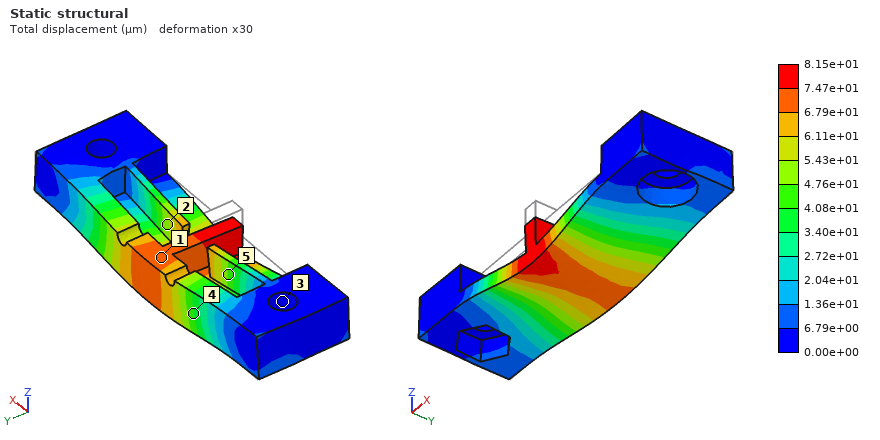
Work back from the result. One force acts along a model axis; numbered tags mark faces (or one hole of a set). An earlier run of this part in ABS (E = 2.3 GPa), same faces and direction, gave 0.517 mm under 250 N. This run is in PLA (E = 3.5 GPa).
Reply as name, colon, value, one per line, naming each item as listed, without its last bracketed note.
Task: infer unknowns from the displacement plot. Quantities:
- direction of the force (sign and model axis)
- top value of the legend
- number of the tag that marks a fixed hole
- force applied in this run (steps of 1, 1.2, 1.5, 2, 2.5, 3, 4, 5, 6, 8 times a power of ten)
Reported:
direction of the force: -Z
top value of the legend: 8.15e+01 µm
number of the tag that marks a fixed hole: 3
force applied in this run: 60 N
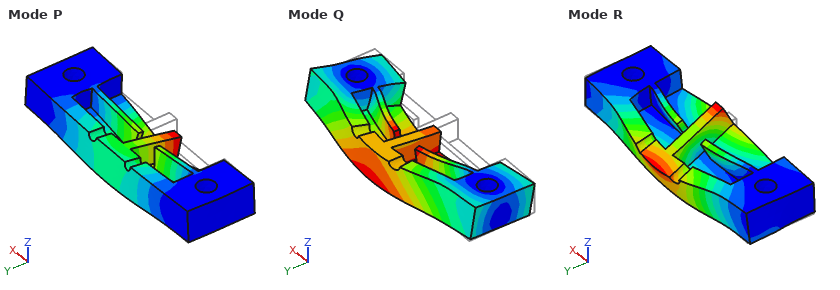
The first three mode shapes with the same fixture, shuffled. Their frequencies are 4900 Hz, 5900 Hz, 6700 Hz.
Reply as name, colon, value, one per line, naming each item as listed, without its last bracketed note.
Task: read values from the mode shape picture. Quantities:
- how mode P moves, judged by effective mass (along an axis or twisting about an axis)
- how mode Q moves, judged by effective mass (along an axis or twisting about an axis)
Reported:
how mode P moves, judged by effective mass: along Z
how mode Q moves, judged by effective mass: along Y
